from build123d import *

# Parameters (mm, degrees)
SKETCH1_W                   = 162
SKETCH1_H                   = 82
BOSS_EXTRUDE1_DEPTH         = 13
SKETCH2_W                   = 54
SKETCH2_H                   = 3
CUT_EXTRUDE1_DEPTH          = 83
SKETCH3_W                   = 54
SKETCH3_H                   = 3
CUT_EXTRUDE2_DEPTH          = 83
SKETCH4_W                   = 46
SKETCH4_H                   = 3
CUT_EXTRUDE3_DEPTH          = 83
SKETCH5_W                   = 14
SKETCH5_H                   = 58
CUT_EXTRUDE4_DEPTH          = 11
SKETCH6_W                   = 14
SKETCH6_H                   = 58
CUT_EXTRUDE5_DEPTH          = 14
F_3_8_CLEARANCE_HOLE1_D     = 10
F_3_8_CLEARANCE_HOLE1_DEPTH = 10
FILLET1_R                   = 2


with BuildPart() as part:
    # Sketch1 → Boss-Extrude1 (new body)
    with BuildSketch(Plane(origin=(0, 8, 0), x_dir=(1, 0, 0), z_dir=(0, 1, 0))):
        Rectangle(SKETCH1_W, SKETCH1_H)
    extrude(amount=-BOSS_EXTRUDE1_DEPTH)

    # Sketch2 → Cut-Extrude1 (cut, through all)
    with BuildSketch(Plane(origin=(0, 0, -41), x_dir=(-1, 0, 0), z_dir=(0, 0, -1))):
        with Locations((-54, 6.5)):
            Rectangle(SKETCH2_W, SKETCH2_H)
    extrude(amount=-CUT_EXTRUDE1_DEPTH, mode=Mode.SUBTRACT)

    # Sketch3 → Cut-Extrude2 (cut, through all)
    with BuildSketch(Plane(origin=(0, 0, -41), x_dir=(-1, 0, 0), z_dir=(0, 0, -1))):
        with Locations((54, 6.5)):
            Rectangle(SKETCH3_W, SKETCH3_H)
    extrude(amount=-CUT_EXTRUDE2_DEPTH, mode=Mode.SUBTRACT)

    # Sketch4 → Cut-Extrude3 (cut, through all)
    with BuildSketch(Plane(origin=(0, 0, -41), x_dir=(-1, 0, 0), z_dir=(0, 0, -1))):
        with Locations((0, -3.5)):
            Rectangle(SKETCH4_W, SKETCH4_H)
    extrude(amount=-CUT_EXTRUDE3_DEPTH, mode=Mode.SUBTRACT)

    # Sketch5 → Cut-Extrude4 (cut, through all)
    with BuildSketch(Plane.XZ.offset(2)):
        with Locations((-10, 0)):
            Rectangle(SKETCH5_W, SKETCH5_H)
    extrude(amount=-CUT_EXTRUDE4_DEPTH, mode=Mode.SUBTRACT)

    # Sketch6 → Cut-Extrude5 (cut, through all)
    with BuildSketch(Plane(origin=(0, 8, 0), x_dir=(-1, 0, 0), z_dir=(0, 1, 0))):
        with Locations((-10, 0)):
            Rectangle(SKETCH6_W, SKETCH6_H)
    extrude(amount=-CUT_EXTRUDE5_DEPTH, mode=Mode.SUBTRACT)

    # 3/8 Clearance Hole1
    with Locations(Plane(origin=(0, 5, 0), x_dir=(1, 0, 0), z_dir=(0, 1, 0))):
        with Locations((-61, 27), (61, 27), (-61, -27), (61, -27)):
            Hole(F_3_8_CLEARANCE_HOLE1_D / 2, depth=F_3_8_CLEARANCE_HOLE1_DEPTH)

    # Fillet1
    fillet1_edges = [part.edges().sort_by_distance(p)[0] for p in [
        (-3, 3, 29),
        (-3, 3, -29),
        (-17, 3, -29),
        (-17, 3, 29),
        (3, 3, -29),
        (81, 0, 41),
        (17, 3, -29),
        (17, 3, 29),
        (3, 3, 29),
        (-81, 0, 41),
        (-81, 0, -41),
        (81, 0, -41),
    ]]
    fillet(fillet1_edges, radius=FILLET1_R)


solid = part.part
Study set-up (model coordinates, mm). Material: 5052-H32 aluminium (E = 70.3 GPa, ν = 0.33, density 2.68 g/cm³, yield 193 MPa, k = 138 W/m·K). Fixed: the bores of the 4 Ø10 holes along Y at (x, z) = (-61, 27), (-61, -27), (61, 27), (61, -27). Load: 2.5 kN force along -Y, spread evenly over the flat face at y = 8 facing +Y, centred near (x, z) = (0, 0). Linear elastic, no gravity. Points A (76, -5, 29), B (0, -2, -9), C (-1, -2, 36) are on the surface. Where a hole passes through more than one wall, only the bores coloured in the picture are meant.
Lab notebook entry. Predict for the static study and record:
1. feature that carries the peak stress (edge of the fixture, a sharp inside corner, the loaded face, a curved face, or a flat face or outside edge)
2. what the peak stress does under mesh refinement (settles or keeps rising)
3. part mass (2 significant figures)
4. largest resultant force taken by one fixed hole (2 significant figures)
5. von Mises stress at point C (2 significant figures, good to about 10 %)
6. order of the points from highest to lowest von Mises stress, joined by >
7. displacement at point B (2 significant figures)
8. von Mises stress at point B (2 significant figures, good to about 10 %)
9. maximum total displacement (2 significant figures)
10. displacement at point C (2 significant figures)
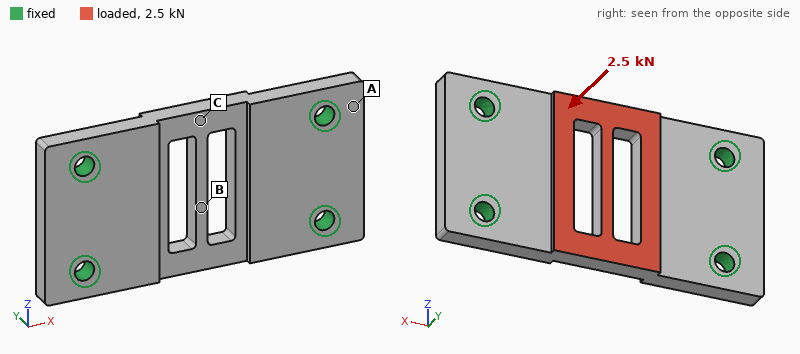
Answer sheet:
edge of the fixture
keeps rising
310 g
960 N
22 MPa
C > B > A
71 µm
14 MPa
73 µm
55 µm
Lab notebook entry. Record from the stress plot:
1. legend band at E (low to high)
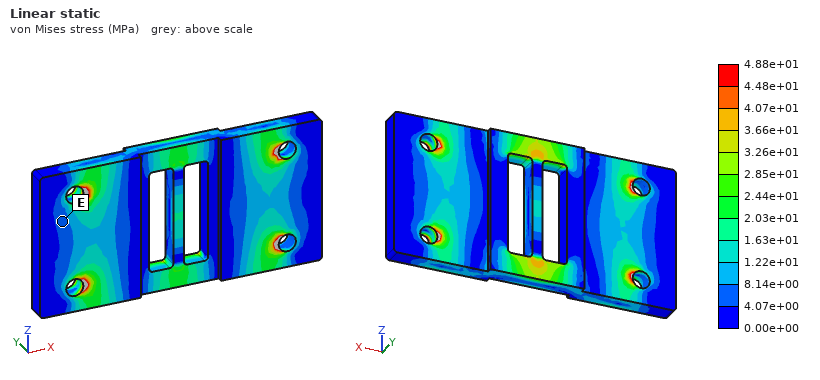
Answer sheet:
4.07e+00 to 8.14e+00 MPa
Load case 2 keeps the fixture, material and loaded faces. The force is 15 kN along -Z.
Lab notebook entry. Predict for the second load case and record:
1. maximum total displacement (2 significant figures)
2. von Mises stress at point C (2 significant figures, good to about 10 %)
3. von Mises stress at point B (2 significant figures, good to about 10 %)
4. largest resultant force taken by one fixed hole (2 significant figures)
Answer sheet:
0.10 mm
45 MPa
9.6 MPa
5.5 kN
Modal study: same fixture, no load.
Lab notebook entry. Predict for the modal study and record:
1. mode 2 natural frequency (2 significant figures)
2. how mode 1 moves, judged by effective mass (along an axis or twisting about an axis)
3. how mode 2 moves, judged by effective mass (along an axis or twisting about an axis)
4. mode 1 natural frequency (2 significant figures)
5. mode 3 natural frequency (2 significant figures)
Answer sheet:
5000 Hz
along Y
twisting about X
3600 Hz
6400 Hz
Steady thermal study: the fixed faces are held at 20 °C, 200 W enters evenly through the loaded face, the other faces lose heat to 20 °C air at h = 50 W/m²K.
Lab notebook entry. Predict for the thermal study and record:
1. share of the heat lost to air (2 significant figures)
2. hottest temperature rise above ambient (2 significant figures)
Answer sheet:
13 %
73 K
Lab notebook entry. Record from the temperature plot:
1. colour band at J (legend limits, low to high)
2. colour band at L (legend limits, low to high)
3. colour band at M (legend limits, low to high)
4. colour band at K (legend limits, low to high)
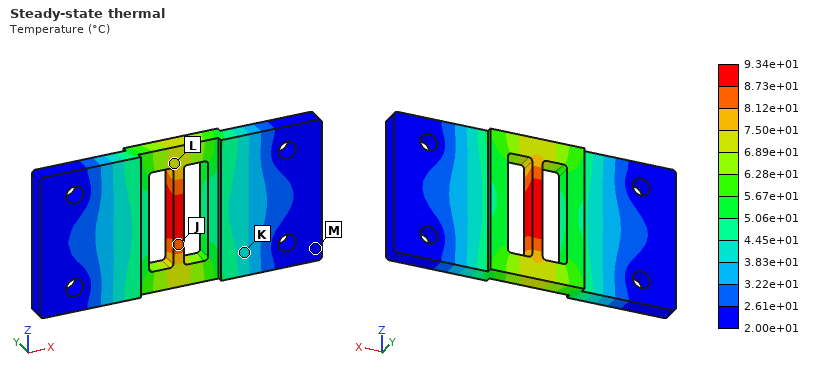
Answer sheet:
8.12e+01 to 8.73e+01 °C
6.89e+01 to 7.50e+01 °C
2.00e+01 to 2.61e+01 °C
3.83e+01 to 4.45e+01 °C
